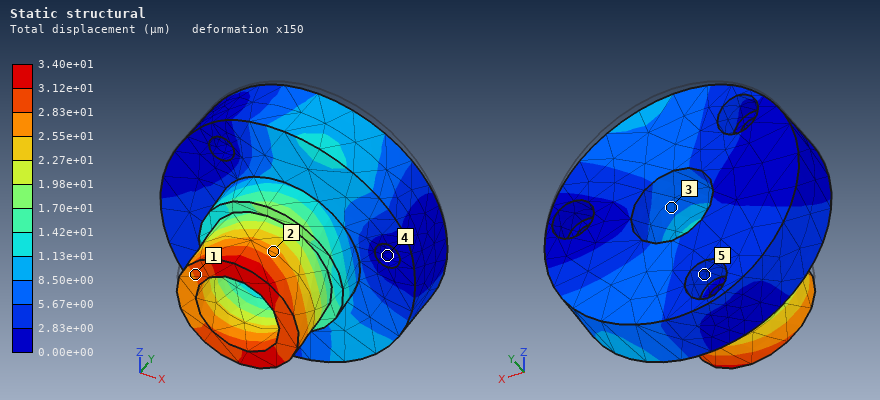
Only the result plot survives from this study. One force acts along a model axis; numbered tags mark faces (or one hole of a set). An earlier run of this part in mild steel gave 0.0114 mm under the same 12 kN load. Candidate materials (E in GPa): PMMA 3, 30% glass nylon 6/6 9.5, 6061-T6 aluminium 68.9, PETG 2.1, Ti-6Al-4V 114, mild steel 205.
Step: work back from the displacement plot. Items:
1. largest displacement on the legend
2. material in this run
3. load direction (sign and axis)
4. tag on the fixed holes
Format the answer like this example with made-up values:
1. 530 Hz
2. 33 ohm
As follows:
1. 3.40e+01 µm
2. 6061-T6 aluminium
3. -Z
4. 4
